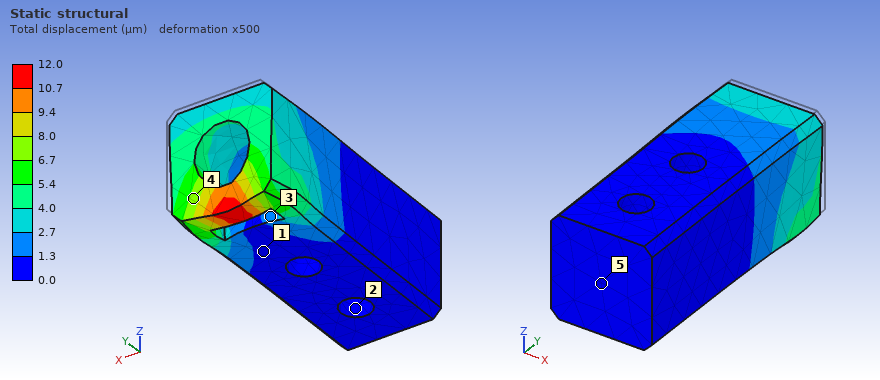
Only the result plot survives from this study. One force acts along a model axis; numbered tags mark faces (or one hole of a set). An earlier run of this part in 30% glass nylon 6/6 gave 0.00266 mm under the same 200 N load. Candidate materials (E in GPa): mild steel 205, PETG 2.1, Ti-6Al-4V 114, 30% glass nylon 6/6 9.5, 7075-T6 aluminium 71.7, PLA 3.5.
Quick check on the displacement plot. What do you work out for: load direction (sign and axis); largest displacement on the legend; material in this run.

-Y
12.0 µm
PETG
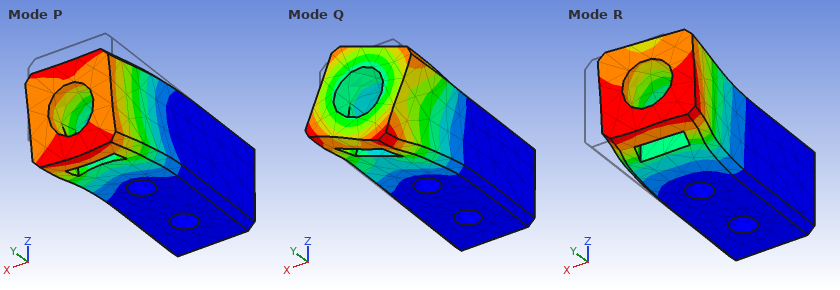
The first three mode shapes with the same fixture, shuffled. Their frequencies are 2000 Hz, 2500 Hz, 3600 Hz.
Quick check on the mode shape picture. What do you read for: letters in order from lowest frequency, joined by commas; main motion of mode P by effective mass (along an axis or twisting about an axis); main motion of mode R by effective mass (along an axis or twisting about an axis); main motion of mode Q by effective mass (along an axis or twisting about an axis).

R, P, Q
along Z
along X
twisting about Y
